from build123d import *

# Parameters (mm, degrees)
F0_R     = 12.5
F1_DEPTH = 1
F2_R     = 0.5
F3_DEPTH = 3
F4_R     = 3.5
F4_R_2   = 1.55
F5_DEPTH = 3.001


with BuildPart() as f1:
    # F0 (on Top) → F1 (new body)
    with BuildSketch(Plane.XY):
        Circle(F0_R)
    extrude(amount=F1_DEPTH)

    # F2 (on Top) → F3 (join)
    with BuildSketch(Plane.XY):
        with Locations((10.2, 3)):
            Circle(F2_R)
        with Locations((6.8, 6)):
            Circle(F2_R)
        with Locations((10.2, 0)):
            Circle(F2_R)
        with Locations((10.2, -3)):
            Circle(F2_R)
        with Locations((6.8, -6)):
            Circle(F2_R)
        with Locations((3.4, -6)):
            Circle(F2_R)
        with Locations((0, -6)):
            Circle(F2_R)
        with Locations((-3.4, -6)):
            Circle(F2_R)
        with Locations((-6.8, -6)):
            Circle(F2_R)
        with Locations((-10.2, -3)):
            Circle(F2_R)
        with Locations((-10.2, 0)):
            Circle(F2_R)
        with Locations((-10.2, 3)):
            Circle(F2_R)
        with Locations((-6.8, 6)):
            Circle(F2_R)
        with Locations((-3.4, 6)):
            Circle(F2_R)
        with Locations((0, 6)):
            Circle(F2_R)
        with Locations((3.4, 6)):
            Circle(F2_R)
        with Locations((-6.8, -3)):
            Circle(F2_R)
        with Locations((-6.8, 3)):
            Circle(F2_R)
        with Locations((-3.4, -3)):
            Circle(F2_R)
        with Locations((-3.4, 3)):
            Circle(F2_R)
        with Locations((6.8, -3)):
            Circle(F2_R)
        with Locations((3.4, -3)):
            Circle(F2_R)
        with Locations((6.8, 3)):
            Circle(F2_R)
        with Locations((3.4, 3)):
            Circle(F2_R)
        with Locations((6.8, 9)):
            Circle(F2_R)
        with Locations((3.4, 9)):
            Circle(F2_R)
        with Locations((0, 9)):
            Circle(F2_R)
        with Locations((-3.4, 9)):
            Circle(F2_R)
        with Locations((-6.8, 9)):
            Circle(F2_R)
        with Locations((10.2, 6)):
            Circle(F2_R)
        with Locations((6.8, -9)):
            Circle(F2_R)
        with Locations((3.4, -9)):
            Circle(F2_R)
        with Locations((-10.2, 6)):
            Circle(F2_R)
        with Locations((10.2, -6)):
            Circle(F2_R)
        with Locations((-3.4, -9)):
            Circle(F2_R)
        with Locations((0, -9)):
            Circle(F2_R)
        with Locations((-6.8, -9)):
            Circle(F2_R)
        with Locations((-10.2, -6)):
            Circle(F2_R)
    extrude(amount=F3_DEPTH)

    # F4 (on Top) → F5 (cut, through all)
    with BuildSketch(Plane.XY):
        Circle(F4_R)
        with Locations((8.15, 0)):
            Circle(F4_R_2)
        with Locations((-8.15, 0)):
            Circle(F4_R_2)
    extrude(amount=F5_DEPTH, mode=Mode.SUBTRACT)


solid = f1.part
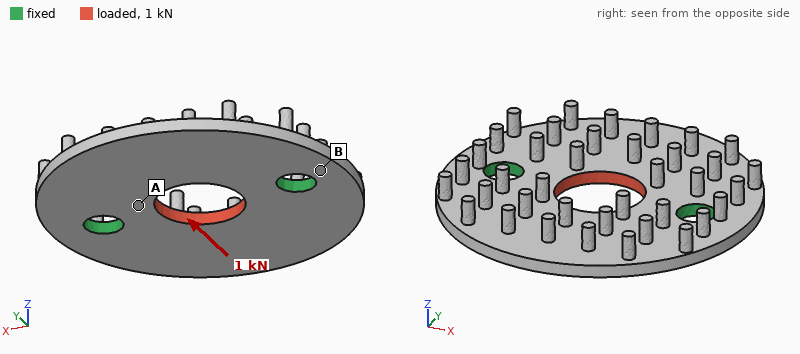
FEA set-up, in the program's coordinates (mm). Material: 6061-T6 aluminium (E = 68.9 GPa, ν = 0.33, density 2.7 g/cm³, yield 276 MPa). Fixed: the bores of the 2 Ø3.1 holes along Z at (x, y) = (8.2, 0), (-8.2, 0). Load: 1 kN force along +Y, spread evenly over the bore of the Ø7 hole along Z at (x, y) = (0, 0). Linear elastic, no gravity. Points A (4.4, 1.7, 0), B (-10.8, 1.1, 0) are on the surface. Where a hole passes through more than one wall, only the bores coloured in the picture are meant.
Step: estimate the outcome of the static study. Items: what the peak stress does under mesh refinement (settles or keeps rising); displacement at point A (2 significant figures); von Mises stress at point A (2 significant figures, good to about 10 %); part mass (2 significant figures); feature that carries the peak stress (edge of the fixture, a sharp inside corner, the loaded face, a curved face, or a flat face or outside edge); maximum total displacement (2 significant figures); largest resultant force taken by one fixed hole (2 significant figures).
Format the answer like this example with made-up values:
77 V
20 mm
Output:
keeps rising
4.9 µm
61 MPa
1.3 g
edge of the fixture
8.4 µm
500 N
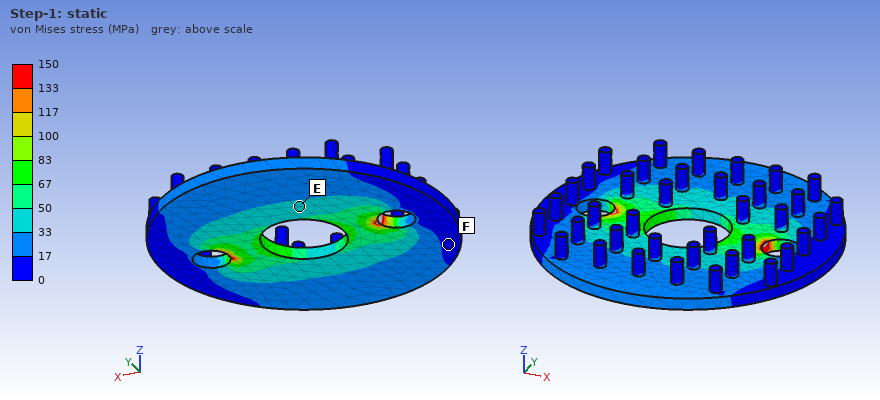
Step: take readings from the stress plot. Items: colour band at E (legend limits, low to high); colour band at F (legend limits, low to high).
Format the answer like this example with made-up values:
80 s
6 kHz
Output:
33 to 50 MPa
0 to 17 MPa
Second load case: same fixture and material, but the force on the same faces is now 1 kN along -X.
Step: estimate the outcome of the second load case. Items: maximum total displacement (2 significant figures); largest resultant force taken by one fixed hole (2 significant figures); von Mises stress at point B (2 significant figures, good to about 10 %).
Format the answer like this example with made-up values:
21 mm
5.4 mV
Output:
6.7 µm
500 N
19 MPa
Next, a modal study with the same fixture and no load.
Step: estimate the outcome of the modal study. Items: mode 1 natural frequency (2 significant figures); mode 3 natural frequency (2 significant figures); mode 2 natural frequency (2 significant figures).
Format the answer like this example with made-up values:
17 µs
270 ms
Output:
6300 Hz
15 kHz
6500 Hz
